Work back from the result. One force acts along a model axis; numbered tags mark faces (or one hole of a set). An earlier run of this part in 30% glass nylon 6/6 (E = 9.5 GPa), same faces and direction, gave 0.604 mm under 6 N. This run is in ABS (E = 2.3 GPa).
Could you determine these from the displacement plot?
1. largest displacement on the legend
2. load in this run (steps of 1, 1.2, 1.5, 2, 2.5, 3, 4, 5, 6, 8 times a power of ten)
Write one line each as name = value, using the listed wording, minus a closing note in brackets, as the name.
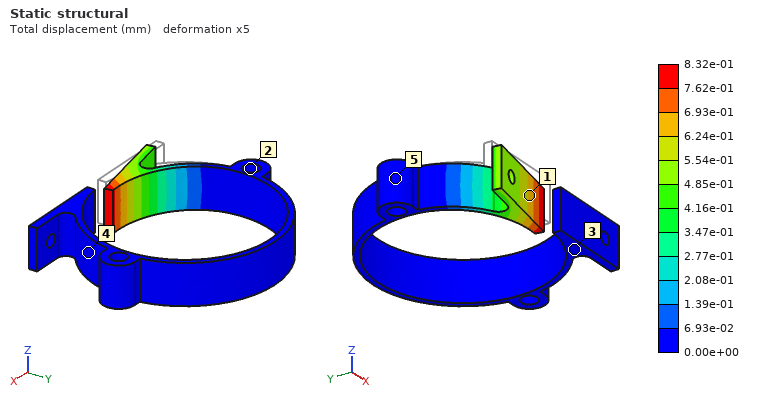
largest displacement on the legend = 8.32e-01 mm
load in this run = 2 N
